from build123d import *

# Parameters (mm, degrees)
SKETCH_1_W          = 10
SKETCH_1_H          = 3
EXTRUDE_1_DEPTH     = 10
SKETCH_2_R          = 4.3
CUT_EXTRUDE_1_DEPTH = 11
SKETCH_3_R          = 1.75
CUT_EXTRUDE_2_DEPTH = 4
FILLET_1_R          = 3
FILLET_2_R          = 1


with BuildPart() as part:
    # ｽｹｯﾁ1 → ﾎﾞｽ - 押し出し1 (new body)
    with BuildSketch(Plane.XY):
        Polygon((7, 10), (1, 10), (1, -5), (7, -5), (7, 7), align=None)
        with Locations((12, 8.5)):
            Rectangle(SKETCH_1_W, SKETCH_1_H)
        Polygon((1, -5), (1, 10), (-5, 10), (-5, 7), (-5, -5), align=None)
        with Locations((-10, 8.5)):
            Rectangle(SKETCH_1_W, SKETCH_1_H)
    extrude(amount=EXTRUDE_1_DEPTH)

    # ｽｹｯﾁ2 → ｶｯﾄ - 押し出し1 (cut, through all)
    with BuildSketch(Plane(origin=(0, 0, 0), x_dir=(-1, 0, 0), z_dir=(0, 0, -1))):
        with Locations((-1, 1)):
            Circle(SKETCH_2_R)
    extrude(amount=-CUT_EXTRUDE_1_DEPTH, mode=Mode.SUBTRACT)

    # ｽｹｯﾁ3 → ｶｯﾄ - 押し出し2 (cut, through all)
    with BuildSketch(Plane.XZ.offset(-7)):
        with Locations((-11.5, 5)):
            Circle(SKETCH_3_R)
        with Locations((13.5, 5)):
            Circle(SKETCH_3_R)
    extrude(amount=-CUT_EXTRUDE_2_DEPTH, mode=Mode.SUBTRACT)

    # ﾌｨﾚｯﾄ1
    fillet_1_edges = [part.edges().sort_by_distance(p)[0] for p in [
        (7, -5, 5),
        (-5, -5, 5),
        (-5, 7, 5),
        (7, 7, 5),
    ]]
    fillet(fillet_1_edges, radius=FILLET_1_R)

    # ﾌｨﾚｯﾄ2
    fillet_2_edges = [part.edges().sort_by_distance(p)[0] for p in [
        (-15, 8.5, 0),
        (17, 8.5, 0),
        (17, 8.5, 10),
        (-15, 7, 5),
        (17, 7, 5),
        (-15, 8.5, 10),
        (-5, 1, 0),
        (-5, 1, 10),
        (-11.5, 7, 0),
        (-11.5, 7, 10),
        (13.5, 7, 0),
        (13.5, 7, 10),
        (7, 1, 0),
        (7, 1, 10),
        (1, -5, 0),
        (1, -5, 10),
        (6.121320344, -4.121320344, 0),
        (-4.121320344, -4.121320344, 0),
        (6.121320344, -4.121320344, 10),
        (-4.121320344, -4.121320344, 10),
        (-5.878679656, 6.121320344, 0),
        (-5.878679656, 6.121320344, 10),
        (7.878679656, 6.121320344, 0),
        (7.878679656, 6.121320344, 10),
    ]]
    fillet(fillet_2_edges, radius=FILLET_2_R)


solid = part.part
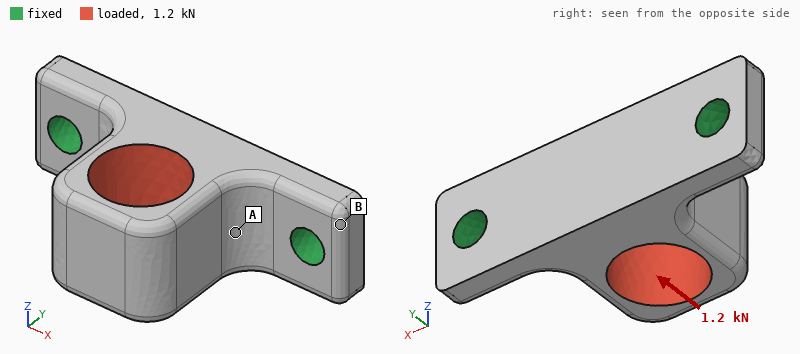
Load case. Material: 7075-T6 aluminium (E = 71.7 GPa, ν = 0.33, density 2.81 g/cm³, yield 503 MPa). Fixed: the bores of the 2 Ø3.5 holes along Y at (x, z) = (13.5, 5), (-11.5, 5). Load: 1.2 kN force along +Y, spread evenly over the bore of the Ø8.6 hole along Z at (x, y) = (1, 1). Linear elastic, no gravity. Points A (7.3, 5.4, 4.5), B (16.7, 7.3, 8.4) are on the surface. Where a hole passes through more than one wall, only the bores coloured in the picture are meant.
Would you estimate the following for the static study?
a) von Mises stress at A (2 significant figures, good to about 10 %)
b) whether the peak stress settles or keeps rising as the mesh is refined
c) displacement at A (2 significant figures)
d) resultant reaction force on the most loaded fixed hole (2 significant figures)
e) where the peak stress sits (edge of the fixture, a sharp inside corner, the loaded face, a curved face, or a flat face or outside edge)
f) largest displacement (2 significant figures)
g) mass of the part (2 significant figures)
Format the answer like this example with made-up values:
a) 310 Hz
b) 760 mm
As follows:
a) 77 MPa
b) keeps rising
c) 12 µm
d) 690 N
e) edge of the fixture
f) 17 µm
g) 4.9 g
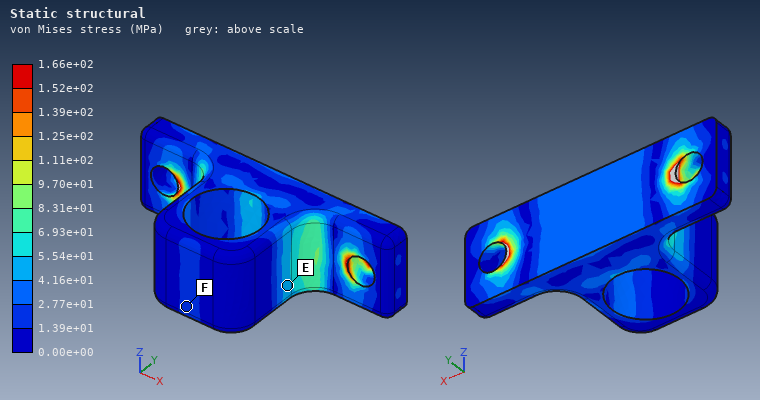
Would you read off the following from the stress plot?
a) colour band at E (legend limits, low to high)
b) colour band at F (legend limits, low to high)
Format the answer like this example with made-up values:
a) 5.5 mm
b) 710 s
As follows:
a) 4.16e+01 to 5.54e+01 MPa
b) 1.39e+01 to 2.77e+01 MPa
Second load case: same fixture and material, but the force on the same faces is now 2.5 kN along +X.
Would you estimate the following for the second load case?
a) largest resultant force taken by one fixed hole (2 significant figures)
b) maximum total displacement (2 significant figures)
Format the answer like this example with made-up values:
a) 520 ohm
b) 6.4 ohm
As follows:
a) 1.6 kN
b) 82 µm
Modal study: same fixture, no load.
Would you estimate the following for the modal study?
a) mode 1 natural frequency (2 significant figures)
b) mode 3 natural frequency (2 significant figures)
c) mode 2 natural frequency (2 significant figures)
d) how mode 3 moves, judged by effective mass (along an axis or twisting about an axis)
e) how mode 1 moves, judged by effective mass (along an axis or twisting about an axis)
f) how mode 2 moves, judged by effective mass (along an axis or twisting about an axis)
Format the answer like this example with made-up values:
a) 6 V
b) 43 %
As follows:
a) 11 kHz
b) 23 kHz
c) 21 kHz
d) along Y
e) along Z
f) along X
